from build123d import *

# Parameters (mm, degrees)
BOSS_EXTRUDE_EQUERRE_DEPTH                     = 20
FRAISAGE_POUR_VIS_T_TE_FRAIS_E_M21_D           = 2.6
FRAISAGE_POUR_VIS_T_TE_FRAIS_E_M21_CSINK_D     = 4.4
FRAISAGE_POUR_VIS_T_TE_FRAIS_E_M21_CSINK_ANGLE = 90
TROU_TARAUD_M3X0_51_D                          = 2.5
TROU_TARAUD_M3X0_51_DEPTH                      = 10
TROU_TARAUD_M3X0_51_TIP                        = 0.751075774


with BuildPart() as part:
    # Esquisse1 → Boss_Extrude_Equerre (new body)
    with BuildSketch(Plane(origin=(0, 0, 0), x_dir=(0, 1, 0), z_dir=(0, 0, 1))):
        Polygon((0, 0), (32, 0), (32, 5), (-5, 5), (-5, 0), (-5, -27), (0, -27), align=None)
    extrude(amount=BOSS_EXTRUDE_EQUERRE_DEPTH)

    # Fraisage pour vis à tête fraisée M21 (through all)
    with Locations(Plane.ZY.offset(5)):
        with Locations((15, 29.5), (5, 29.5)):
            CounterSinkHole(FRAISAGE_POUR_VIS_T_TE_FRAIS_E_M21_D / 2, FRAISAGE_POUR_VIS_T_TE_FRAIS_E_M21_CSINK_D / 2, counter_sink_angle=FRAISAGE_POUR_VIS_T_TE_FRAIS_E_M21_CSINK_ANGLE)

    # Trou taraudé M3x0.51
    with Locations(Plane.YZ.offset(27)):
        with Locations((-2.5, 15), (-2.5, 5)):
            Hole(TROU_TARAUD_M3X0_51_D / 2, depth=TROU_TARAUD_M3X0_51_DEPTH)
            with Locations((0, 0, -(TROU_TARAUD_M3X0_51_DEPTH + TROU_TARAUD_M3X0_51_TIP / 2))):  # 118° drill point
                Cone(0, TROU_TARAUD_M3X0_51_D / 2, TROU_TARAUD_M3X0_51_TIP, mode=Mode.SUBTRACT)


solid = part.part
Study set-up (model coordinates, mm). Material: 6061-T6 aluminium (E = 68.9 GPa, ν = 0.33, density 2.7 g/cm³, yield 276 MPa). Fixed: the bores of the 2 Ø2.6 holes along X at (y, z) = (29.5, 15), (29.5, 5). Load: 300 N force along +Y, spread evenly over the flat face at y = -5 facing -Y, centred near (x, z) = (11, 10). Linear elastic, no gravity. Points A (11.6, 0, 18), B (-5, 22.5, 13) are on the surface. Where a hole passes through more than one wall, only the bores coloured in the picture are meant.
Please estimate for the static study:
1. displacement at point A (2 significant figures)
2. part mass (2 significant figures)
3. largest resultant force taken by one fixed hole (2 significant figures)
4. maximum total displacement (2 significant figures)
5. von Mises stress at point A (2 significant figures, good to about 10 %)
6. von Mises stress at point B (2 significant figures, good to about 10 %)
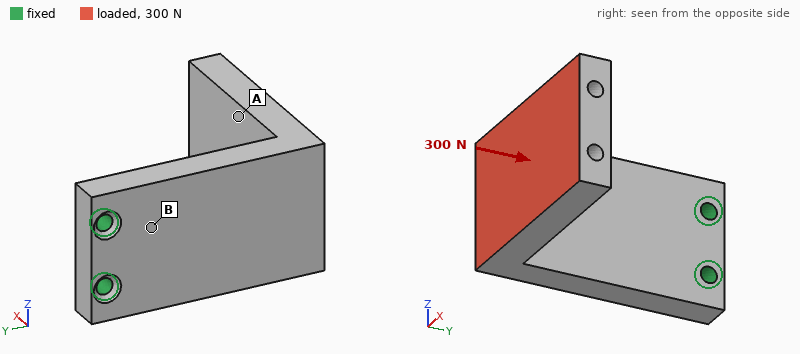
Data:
0.19 mm
17 g
150 N
0.36 mm
13 MPa
43 MPa
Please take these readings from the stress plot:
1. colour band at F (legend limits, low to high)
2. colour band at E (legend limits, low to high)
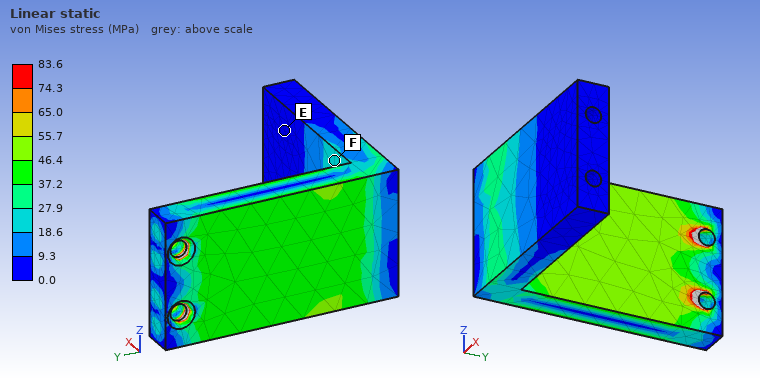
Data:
18.6 to 27.9 MPa
0.0 to 9.3 MPa
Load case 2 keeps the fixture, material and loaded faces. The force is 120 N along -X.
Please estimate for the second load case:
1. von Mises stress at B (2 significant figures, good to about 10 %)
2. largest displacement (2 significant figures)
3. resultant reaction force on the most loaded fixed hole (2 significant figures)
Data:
37 MPa
0.20 mm
61 N
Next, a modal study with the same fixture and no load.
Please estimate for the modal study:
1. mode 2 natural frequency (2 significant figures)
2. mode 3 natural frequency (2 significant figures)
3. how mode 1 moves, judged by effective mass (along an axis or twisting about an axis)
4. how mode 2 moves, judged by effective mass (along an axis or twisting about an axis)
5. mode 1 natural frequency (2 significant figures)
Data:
2500 Hz
4200 Hz
along X
along Z
1400 Hz
